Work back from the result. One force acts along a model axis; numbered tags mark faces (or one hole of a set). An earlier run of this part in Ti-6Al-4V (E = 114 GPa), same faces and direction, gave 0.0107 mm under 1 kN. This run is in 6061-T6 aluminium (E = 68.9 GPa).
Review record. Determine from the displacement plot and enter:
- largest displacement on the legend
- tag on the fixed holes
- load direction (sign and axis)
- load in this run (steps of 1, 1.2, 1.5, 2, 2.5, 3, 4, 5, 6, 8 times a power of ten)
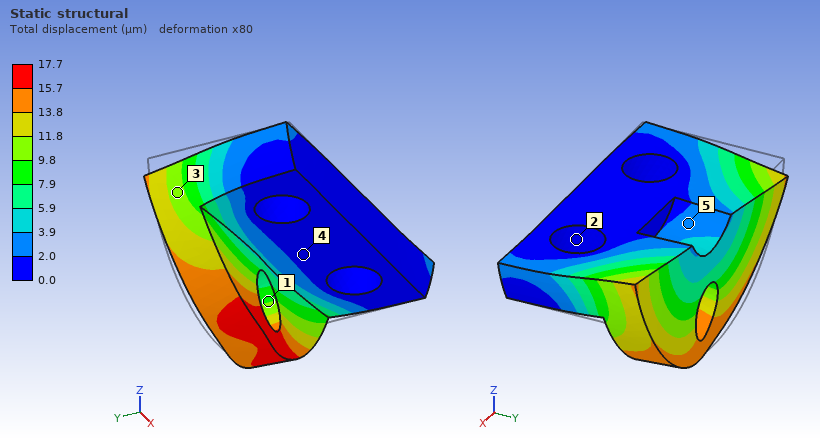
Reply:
17.7 µm
2
+X
1 kN
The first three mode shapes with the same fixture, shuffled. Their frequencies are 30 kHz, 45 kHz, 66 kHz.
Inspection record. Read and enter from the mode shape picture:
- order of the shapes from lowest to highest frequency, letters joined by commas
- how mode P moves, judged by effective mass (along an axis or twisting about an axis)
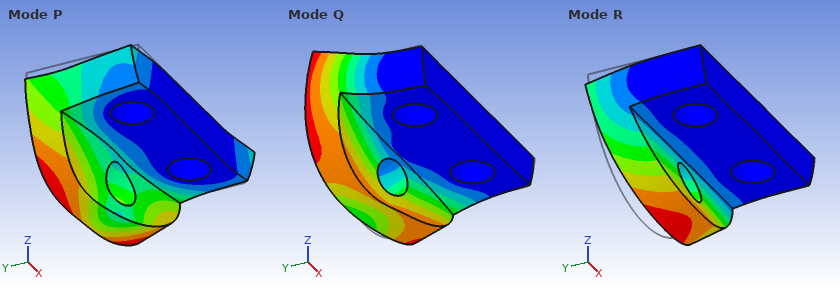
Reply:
R, Q, P
along X
